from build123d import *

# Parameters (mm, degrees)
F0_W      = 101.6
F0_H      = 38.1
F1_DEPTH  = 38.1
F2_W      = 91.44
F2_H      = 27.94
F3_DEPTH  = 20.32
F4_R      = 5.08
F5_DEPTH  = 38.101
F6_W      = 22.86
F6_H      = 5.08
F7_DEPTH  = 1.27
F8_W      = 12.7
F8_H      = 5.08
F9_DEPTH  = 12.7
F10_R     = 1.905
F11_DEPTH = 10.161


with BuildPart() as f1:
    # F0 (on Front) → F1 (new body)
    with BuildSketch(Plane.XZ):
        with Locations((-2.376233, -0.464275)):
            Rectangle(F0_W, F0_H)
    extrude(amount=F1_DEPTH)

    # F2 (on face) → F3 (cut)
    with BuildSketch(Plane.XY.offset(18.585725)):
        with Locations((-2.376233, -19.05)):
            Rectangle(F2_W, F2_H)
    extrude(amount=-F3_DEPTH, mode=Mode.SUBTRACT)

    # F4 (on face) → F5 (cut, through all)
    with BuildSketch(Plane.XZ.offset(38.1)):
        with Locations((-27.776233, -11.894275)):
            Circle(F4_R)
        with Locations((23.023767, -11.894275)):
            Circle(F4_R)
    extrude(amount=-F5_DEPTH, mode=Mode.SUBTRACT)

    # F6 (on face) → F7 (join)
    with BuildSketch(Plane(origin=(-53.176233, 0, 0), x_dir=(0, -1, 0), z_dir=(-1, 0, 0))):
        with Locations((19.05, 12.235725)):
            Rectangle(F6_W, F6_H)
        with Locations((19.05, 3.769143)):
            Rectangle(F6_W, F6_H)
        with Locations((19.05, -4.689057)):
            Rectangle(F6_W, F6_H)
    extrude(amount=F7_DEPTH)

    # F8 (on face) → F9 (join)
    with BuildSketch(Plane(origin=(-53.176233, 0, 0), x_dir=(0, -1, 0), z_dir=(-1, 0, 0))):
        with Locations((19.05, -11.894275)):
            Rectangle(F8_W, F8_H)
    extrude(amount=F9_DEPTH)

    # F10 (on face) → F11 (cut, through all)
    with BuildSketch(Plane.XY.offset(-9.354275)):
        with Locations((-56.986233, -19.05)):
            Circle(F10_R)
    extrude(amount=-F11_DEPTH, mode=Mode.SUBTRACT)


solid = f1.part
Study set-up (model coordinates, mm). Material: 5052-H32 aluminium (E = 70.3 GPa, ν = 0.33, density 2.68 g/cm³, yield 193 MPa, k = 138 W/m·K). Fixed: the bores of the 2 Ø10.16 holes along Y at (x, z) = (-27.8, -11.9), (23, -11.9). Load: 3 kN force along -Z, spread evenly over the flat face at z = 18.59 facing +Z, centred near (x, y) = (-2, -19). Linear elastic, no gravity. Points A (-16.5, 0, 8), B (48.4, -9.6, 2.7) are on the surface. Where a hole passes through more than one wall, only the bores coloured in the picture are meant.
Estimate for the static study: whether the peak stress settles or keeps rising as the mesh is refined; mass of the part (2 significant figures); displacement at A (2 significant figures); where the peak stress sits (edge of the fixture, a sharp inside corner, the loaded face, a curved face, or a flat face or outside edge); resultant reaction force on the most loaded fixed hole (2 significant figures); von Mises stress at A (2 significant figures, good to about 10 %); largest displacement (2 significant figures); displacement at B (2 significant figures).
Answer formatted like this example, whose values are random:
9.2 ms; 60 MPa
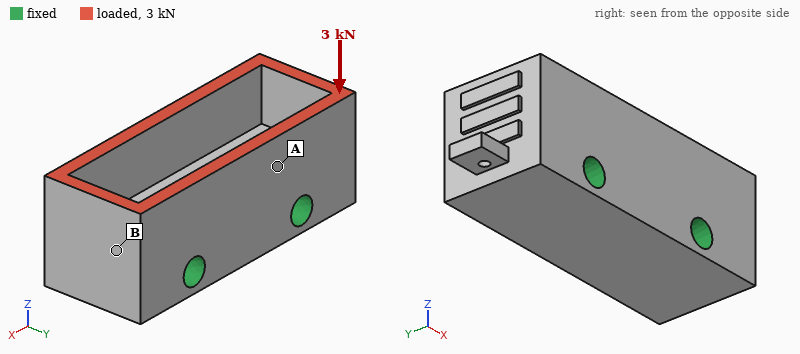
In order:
keeps rising; 240 g; 0.91 µm; edge of the fixture; 1.5 kN; 2.7 MPa; 2.8 µm; 2.1 µm
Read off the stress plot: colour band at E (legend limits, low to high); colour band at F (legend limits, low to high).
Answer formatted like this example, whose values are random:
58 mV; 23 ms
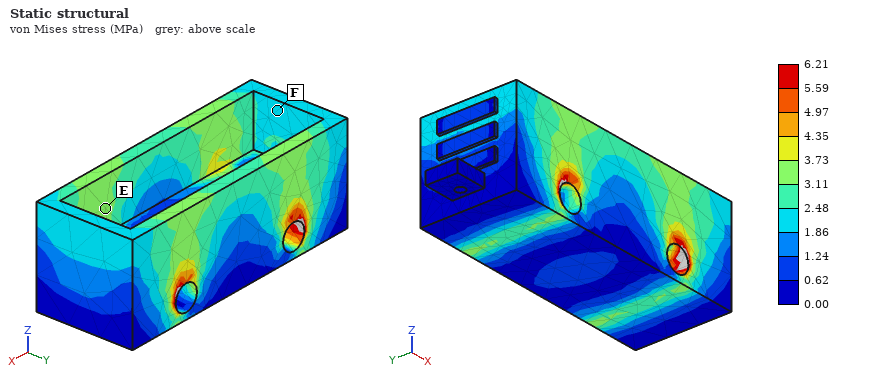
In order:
3.11 to 3.73 MPa; 1.86 to 2.48 MPa
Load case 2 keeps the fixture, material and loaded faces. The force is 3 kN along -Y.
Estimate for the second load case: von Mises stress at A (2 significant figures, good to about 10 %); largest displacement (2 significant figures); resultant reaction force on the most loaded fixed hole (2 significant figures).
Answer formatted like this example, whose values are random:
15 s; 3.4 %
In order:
23 MPa; 54 µm; 1.5 kN
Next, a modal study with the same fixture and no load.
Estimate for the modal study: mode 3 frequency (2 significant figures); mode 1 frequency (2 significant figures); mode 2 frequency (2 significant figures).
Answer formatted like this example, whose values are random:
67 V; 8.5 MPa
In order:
11 kHz; 9000 Hz; 9100 Hz
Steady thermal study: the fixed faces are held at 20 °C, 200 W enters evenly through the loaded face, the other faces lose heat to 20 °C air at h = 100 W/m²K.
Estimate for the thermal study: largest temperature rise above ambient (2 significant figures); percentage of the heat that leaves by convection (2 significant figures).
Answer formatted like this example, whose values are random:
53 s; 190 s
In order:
31 K; 12 %
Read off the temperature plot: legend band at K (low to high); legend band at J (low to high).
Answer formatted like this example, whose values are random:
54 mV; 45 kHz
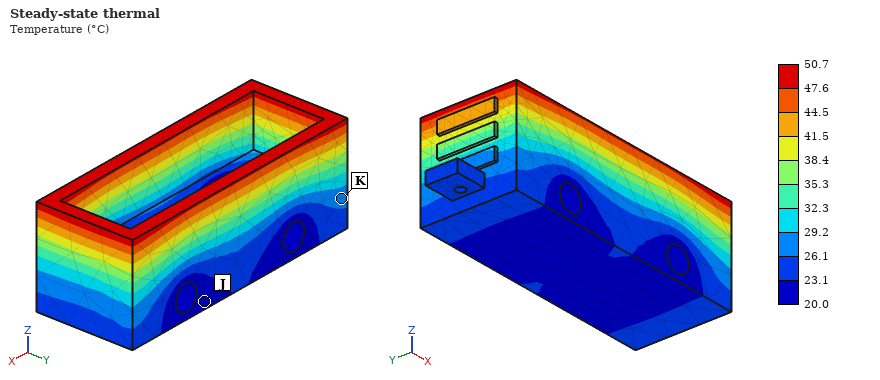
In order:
26.1 to 29.2 °C; 20.0 to 23.1 °C
